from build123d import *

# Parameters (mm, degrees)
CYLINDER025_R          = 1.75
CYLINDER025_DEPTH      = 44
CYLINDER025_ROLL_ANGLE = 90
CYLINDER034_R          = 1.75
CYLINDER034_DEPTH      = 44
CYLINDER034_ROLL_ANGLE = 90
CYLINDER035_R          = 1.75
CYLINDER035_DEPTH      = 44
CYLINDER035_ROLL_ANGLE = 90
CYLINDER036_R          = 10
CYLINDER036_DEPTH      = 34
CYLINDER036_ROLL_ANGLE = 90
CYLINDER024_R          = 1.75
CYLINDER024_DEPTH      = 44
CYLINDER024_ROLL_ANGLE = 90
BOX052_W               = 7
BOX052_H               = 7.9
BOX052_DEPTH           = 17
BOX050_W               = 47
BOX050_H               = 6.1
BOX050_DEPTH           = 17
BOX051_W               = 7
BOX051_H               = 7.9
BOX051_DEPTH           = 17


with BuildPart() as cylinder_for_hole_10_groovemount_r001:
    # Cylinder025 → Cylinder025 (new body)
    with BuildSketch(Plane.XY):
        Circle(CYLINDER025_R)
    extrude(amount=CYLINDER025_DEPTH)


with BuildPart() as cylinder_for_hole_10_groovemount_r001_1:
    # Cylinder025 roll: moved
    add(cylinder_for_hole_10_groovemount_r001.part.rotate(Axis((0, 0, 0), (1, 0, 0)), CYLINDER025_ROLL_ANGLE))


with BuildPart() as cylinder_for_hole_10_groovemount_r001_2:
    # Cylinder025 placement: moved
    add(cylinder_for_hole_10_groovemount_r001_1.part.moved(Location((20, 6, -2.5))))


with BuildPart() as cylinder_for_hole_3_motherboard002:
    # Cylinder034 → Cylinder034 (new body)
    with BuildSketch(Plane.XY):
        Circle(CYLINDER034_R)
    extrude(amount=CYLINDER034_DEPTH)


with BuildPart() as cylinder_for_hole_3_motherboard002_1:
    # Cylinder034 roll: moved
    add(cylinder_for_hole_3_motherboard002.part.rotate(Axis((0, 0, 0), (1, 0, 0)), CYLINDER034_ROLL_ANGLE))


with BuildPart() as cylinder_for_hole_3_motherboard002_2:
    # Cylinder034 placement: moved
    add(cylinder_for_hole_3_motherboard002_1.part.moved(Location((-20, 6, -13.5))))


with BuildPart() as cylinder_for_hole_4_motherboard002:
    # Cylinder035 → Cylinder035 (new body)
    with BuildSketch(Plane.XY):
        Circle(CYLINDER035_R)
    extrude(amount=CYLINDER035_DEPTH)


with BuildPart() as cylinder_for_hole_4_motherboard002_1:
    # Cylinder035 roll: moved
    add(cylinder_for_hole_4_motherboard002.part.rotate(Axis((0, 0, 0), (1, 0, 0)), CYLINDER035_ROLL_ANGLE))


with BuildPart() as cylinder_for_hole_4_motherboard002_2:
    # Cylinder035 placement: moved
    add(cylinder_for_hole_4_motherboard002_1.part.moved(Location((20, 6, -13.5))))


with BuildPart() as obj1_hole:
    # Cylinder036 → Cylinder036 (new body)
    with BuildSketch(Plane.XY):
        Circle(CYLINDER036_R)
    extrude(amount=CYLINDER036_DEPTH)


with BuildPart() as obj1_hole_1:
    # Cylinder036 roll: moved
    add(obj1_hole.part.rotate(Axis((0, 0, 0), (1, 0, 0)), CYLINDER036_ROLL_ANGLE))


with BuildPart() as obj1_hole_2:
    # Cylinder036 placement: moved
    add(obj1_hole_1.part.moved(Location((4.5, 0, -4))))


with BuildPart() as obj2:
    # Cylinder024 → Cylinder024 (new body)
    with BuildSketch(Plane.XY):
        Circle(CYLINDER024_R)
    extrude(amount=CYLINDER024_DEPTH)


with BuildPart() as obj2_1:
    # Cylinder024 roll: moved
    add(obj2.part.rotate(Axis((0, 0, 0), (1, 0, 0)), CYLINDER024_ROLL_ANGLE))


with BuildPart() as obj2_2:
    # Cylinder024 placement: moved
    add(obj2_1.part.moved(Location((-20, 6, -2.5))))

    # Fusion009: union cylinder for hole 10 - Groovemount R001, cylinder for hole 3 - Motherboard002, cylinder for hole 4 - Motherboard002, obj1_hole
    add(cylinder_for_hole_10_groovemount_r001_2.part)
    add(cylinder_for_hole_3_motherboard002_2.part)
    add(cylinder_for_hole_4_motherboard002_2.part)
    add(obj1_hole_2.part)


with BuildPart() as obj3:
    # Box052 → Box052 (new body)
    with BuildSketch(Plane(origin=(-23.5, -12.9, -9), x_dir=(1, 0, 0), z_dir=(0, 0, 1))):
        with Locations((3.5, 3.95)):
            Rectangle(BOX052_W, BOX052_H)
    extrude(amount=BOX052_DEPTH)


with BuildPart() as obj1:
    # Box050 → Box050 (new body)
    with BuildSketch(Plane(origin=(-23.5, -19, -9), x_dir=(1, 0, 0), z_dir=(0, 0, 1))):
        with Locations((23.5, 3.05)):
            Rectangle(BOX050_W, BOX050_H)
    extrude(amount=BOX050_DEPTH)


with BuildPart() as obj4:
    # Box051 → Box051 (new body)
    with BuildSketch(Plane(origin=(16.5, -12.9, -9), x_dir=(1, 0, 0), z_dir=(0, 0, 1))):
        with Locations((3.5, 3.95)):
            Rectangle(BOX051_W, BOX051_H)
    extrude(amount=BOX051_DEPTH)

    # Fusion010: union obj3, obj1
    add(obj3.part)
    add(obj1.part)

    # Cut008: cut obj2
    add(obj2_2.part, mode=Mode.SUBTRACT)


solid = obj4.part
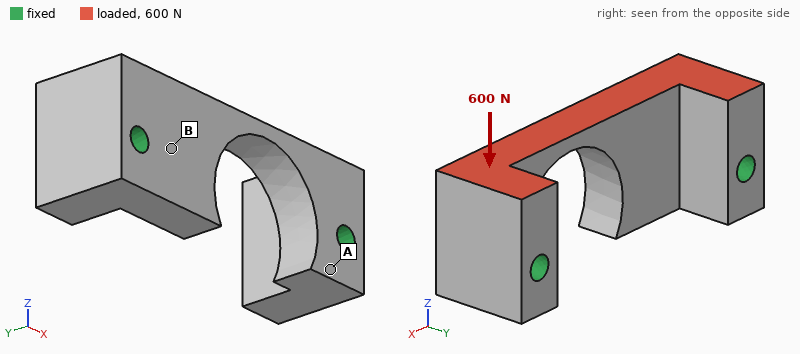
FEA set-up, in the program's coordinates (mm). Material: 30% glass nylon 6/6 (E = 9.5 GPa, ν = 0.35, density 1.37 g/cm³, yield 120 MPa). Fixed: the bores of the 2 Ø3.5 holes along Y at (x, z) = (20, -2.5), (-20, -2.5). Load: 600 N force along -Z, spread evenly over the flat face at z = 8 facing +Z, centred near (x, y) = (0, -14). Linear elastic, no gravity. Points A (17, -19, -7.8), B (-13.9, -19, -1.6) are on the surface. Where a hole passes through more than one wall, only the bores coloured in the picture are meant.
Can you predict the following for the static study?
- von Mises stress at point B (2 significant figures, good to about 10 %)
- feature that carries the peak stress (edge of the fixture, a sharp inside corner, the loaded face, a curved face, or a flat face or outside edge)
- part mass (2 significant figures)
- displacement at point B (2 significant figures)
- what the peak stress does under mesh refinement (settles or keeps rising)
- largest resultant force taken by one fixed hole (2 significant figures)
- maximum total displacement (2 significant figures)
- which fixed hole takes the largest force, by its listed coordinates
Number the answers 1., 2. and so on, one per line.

1. 3.8 MPa
2. edge of the fixture
3. 6.8 g
4. 8.7 µm
5. keeps rising
6. 350 N
7. 34 µm
8. (-20, -2.5)
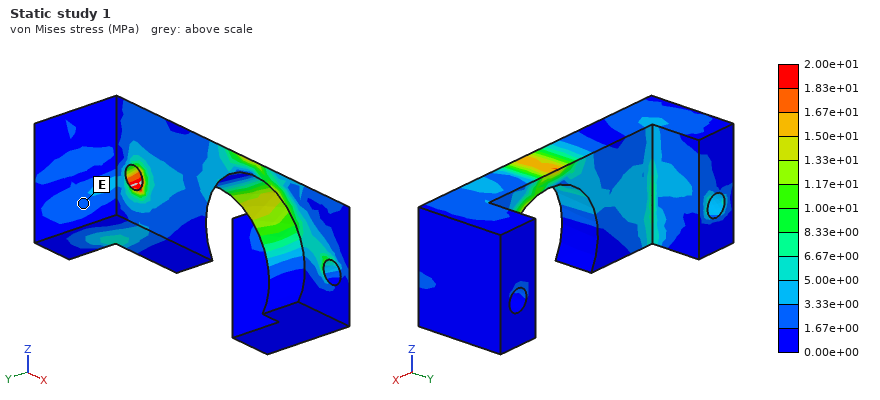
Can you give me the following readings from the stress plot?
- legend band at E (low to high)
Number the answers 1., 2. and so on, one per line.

1. 1.67e+00 to 3.33e+00 MPa
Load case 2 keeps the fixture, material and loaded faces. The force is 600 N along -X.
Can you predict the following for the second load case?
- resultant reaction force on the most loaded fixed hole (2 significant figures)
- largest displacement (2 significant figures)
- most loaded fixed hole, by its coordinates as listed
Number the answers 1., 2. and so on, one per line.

1. 330 N
2. 37 µm
3. (-20, -2.5)
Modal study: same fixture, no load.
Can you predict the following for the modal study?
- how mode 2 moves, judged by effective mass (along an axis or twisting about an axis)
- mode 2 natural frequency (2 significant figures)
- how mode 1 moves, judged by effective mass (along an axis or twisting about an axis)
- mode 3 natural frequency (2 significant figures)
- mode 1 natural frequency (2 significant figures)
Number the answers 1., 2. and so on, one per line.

1. along Z
2. 11 kHz
3. along Y
4. 17 kHz
5. 11 kHz
